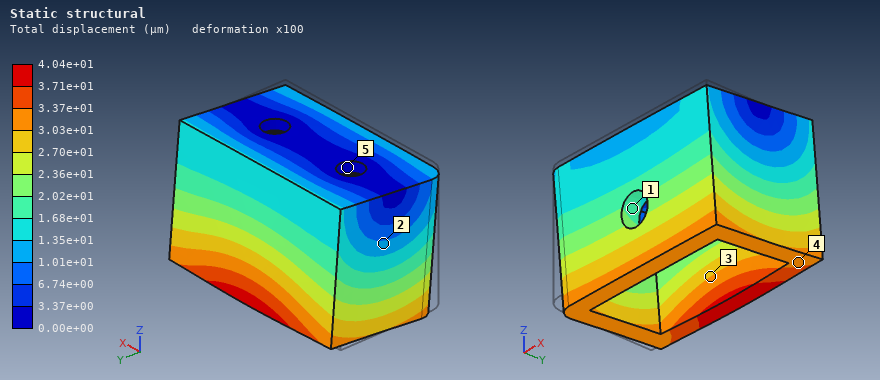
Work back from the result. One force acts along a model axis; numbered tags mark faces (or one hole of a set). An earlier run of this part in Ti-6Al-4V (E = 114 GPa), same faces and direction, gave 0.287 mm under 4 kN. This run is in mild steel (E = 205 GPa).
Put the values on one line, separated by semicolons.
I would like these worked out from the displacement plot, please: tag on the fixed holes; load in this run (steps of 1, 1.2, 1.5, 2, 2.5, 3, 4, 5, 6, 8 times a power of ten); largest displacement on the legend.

5; 1 kN; 4.04e+01 µm
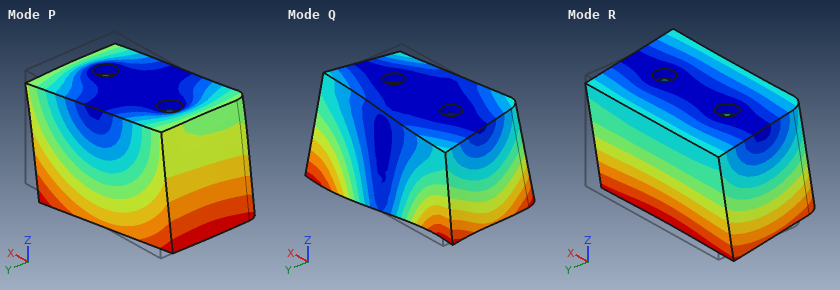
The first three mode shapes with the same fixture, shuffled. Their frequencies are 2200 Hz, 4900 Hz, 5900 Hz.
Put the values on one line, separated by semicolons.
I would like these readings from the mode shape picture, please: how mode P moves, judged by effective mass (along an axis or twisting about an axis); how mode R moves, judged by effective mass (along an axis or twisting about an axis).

along X; along Y
